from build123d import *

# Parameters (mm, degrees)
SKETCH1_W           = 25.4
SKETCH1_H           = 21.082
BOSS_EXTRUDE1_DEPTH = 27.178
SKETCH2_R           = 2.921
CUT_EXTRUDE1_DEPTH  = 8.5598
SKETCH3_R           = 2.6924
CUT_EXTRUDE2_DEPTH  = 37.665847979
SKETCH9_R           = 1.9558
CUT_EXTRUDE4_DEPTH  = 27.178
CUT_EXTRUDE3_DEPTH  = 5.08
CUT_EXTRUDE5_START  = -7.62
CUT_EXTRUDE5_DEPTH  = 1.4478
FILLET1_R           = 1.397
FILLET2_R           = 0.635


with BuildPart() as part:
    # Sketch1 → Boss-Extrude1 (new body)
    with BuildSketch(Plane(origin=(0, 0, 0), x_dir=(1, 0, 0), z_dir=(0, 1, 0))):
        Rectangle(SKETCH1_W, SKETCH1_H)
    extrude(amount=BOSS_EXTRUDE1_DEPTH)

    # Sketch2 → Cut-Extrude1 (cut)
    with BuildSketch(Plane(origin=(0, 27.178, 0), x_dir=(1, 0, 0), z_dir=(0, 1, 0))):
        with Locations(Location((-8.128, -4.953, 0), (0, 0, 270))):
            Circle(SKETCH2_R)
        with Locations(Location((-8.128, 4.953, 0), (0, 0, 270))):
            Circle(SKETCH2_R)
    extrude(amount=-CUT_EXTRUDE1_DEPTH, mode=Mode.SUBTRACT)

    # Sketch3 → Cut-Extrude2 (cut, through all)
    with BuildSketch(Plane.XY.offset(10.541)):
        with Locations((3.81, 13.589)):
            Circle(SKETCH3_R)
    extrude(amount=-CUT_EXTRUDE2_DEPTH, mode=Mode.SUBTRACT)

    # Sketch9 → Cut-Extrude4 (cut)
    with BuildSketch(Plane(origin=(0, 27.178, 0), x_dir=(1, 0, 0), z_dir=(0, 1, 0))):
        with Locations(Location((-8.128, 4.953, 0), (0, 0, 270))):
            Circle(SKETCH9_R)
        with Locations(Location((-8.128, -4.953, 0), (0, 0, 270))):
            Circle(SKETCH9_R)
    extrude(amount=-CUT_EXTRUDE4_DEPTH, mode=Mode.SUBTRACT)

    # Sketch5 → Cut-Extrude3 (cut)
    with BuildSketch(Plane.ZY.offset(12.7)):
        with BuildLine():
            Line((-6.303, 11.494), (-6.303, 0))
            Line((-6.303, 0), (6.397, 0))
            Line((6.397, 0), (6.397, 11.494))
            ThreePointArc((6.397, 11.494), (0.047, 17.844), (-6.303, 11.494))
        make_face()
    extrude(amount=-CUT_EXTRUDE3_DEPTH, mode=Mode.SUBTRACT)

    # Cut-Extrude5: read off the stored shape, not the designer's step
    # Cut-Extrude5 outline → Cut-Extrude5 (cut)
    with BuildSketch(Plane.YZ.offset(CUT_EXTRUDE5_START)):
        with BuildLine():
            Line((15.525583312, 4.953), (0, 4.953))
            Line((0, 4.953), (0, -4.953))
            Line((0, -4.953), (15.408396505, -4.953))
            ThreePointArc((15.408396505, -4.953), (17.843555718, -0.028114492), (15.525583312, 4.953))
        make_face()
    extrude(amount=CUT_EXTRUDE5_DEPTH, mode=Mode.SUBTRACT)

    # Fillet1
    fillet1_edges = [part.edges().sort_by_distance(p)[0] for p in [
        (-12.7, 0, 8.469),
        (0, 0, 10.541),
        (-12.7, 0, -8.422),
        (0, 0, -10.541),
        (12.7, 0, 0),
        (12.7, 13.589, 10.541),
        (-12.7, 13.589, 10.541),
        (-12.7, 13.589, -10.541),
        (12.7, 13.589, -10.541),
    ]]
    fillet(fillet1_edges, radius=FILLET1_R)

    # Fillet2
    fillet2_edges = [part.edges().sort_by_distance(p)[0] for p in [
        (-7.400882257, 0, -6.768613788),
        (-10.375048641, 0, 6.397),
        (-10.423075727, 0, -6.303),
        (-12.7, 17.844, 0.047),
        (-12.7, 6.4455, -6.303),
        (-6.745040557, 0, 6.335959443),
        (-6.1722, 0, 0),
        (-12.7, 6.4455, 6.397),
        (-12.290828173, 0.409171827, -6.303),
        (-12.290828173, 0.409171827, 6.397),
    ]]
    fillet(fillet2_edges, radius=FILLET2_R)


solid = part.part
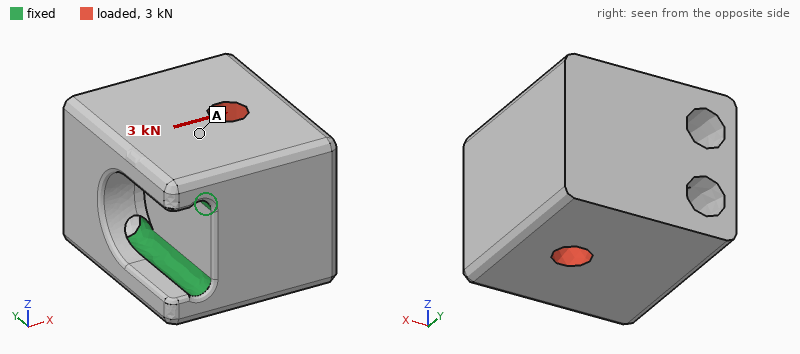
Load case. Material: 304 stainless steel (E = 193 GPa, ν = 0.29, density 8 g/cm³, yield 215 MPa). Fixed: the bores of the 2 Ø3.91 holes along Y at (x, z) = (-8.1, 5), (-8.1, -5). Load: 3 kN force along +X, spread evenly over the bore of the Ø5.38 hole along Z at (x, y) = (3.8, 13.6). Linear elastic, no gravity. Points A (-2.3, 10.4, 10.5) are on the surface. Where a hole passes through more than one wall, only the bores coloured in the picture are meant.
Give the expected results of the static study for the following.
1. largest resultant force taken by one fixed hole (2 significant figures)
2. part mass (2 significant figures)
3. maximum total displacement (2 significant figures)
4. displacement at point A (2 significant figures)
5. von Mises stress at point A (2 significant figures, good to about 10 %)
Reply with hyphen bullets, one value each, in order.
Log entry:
- 1.5 kN
- 96 g
- 1.2 µm
- 0.36 µm
- 8.2 MPa
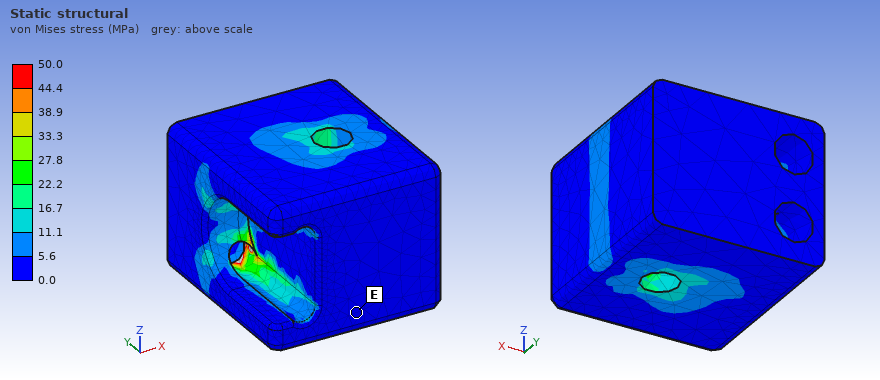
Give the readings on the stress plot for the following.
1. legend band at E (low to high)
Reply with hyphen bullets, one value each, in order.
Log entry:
- 0.0 to 5.6 MPa
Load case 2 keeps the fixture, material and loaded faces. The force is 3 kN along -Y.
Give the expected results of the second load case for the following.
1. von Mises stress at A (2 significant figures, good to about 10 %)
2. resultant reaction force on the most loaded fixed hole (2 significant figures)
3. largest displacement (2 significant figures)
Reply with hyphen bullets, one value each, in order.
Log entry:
- 19 MPa
- 1.5 kN
- 4.5 µm
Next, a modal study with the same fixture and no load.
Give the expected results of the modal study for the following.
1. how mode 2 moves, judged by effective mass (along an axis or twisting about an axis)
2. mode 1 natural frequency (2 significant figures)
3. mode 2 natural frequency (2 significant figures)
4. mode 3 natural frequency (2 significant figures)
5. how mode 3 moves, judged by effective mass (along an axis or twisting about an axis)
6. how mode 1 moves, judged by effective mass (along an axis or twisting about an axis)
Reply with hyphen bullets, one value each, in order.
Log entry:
- along Z
- 17 kHz
- 18 kHz
- 27 kHz
- twisting about X
- along Y
